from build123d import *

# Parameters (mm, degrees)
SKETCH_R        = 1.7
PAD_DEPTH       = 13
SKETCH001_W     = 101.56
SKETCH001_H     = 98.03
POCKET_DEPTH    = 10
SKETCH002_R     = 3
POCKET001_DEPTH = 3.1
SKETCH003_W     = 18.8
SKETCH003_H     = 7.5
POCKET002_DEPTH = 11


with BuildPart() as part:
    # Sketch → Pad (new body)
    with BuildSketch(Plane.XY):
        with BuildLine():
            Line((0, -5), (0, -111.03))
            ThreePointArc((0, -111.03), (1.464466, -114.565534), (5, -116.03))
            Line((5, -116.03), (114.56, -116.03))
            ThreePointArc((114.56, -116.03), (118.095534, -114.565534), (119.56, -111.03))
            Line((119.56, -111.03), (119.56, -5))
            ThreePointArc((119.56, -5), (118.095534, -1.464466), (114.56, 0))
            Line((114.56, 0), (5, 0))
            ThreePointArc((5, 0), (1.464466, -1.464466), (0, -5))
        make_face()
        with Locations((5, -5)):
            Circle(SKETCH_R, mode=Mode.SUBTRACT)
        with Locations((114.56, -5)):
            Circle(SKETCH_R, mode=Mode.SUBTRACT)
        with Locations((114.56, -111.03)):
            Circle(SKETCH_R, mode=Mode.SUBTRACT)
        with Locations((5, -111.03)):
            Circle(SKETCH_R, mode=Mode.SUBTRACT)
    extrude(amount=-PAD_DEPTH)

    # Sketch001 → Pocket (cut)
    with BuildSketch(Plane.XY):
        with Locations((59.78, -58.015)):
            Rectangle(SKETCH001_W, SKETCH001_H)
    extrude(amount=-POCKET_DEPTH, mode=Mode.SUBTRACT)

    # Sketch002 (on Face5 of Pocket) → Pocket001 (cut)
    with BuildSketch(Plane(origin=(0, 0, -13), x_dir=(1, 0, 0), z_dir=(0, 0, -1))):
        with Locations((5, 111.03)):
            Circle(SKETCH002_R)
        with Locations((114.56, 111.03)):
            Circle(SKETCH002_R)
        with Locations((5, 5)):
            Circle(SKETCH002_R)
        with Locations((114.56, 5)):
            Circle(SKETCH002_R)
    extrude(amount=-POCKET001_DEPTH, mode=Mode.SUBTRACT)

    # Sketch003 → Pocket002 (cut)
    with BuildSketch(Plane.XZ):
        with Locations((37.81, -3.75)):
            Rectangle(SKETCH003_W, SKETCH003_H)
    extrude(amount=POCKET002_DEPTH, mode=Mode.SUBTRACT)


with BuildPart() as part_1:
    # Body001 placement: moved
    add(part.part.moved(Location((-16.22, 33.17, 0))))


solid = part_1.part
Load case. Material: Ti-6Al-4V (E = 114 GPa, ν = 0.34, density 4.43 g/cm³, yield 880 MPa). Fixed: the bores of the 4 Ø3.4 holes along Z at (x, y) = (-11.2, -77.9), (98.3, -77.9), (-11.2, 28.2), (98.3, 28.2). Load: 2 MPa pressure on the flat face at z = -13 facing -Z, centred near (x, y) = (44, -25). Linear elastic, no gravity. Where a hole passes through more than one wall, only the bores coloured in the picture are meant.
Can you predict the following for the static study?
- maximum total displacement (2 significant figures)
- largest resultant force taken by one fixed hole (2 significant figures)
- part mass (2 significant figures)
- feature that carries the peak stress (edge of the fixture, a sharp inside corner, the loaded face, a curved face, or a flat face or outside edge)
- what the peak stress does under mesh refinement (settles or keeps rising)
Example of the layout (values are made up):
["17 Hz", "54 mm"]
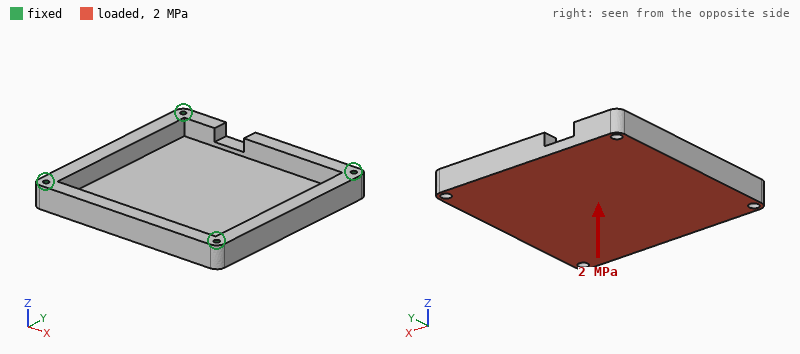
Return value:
["1.5 mm", "12 kN", "350 g", "edge of the fixture", "keeps rising"]
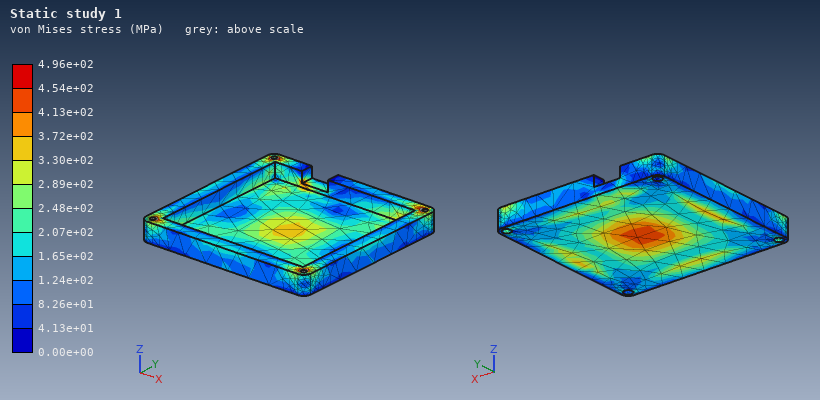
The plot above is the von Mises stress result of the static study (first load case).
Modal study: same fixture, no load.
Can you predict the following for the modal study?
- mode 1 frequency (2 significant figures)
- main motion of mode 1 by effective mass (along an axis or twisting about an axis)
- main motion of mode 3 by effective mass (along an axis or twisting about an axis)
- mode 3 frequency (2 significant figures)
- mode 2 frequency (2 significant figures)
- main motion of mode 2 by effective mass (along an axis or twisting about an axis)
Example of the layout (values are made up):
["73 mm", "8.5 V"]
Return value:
["2000 Hz", "along Z", "twisting about Y", "3700 Hz", "3600 Hz", "twisting about X"]
